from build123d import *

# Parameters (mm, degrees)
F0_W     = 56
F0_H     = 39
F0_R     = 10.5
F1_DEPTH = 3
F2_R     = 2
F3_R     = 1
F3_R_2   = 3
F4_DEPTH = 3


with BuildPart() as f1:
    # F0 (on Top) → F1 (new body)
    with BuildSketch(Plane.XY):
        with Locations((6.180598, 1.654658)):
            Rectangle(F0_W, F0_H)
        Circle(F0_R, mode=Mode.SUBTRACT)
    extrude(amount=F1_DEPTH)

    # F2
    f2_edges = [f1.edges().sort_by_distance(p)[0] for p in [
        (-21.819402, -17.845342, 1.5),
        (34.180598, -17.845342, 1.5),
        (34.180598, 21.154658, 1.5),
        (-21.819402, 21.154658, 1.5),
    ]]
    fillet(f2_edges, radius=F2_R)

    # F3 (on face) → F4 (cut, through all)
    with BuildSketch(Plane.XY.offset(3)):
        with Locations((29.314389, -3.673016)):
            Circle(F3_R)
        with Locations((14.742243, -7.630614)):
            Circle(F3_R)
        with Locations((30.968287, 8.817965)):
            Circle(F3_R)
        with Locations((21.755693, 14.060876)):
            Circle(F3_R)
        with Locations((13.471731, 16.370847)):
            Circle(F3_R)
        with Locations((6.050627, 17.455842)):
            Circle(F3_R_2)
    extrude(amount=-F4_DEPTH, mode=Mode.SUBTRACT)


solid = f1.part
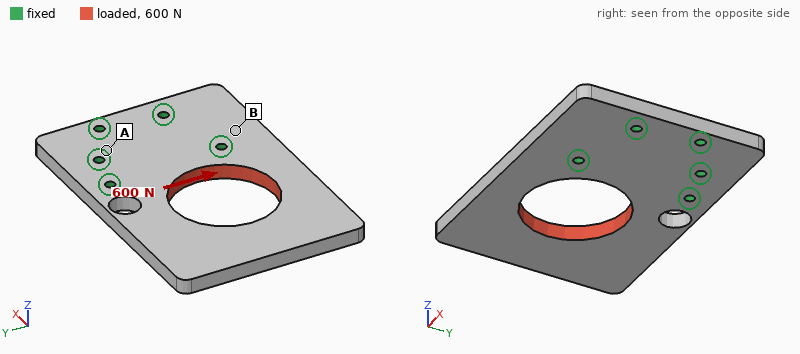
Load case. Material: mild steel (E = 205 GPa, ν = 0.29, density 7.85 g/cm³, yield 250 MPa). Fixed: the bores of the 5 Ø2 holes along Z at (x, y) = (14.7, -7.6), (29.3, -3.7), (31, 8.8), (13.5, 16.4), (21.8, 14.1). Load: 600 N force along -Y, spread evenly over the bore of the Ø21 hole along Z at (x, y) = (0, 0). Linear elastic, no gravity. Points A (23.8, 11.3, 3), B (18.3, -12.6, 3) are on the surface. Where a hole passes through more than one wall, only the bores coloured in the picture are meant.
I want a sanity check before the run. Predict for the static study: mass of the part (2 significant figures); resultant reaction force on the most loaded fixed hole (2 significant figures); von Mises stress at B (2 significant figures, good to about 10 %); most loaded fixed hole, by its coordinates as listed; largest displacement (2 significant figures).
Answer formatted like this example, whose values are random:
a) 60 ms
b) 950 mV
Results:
a) 42 g
b) 450 N
c) 13 MPa
d) (14.7, -7.6)
e) 8.9 µm
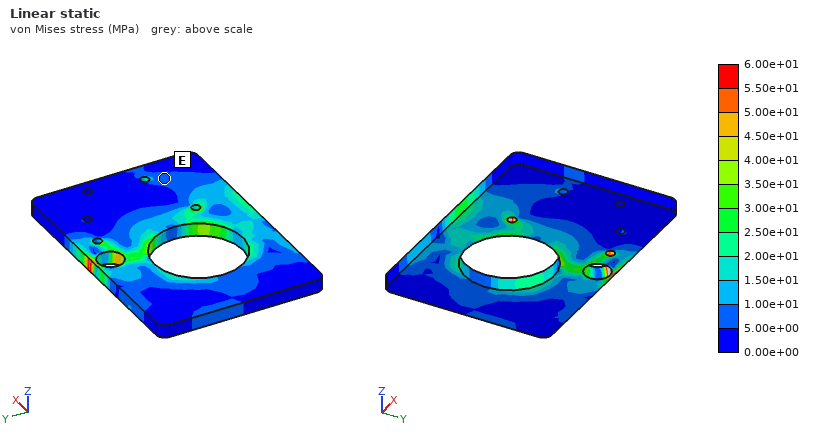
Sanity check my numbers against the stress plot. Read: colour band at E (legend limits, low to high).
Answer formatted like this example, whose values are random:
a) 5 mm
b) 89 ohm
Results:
a) 5.00e+00 to 1.00e+01 MPa
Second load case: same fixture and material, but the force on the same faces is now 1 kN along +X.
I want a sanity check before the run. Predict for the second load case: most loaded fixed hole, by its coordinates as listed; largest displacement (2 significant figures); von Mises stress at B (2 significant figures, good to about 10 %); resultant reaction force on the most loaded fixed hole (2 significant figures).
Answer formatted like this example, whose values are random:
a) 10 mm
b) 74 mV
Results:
a) (14.7, -7.6)
b) 3.2 µm
c) 11 MPa
d) 470 N
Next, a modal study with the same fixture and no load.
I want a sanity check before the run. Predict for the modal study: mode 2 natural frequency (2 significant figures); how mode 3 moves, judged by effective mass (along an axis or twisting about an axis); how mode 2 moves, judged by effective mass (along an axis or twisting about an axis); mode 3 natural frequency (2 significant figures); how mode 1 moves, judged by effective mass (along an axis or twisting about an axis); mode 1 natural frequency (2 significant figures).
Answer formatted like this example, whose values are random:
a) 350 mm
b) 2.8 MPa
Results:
a) 3400 Hz
b) along Y
c) twisting about X
d) 8000 Hz
e) along Z
f) 1400 Hz
